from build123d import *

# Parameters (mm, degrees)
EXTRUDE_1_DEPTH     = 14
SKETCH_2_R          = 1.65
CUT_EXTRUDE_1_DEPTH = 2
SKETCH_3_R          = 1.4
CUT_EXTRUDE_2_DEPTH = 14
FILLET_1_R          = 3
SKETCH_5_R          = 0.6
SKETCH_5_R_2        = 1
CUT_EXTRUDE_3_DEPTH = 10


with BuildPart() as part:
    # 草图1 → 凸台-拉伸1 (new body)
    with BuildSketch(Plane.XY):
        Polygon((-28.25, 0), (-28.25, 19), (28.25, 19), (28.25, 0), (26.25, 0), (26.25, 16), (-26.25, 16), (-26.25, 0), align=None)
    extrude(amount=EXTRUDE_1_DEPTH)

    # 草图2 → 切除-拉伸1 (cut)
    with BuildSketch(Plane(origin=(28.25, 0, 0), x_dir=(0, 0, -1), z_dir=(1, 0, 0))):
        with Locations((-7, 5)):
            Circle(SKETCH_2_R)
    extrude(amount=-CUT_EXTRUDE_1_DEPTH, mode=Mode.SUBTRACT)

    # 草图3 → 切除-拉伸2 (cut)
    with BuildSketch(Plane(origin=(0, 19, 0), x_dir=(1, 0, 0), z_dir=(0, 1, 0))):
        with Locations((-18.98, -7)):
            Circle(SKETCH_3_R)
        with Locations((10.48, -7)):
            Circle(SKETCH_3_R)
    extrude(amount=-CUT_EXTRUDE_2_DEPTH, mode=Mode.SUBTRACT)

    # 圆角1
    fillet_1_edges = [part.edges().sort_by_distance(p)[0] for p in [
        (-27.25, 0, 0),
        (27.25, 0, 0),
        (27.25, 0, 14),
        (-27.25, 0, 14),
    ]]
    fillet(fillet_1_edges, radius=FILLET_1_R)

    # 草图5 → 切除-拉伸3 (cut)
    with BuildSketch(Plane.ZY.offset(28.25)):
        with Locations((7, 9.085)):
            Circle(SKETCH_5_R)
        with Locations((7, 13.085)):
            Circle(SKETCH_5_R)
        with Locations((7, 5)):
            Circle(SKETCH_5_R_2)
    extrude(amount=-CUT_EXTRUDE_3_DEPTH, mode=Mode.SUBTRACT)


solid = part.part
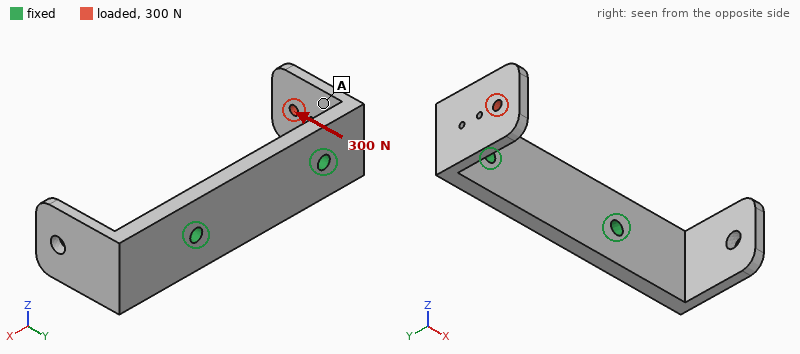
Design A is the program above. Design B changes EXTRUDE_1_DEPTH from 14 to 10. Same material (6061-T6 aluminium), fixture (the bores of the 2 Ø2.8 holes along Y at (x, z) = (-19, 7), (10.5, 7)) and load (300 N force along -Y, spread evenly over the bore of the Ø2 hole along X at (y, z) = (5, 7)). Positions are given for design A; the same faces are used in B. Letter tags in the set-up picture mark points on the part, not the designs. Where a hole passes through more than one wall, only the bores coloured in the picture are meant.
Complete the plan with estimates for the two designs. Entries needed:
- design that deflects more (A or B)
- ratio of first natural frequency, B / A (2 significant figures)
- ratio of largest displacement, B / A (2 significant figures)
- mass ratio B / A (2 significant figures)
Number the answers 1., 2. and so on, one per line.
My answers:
1. B
2. 1.0
3. 1.3
4. 0.71
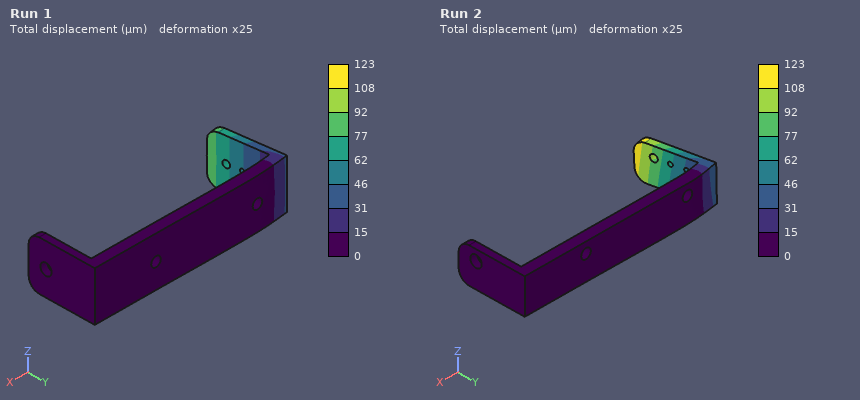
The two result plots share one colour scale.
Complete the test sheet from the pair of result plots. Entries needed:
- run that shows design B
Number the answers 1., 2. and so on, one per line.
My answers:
1. Run 2
